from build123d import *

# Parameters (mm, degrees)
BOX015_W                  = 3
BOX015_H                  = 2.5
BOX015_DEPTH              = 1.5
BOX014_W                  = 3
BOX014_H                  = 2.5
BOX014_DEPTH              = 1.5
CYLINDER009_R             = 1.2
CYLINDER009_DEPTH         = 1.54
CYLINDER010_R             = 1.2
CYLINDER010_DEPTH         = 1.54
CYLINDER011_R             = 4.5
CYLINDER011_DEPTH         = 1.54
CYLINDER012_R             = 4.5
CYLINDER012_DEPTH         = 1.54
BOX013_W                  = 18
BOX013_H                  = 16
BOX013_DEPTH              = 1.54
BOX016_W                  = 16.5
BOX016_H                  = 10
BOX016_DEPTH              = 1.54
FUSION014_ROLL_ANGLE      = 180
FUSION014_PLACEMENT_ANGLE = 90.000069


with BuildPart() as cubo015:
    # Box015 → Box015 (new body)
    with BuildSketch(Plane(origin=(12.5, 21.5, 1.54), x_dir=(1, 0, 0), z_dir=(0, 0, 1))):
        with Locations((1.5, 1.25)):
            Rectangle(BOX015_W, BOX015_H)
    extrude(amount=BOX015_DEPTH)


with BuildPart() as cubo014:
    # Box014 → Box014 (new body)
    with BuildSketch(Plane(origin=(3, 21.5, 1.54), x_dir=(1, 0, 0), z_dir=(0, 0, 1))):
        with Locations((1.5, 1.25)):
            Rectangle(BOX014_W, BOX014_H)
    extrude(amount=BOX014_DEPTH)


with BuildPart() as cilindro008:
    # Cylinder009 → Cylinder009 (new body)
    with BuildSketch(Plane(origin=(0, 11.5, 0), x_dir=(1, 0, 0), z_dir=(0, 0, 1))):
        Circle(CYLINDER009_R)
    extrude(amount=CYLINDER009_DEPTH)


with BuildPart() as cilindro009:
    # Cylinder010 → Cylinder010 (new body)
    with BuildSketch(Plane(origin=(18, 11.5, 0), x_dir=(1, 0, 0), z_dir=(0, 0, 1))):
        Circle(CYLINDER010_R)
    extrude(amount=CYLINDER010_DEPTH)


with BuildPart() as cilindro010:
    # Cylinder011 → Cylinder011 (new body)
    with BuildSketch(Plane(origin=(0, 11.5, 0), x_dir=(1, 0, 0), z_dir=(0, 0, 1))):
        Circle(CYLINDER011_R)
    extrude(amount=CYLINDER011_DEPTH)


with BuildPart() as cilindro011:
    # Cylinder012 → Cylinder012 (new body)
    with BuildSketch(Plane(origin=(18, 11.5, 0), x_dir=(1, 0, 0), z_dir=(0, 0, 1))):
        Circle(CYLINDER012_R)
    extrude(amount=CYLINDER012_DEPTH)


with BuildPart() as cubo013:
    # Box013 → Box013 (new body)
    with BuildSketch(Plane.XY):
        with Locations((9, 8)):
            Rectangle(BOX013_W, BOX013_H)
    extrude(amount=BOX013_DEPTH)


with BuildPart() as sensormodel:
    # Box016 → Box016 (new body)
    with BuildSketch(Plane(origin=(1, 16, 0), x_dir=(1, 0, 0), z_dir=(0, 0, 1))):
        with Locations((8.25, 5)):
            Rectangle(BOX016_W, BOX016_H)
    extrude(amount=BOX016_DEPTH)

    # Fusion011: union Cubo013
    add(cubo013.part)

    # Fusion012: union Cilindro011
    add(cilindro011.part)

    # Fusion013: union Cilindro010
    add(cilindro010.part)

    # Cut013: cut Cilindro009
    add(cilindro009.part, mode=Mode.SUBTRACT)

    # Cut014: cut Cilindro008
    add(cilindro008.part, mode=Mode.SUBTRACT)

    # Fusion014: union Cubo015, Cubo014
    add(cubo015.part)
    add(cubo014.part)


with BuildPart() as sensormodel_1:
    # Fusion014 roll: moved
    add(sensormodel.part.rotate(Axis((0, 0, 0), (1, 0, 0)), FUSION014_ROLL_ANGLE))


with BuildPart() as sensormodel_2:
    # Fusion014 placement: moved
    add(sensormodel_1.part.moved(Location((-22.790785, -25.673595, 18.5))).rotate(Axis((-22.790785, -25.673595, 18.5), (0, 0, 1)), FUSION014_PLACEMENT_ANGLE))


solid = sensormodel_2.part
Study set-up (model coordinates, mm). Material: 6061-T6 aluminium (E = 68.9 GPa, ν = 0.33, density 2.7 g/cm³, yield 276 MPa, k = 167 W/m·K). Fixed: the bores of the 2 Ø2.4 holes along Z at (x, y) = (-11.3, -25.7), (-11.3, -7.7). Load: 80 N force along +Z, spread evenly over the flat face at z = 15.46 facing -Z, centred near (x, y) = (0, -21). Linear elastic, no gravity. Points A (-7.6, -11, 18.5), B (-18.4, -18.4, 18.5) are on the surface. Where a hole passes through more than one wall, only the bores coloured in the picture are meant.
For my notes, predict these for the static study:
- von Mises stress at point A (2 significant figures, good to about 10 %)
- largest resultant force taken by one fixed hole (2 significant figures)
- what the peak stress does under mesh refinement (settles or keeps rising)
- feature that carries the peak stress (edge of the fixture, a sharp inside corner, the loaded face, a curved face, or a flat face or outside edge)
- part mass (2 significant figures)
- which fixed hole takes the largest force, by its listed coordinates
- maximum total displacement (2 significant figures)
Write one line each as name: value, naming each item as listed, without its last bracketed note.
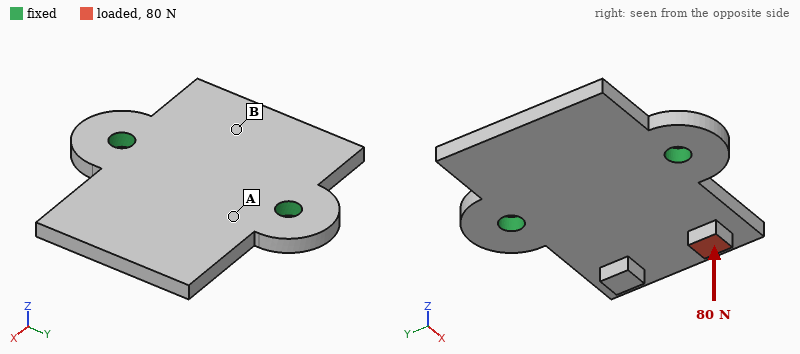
von Mises stress at point A: 73 MPa
largest resultant force taken by one fixed hole: 64 N
what the peak stress does under mesh refinement: keeps rising
feature that carries the peak stress: edge of the fixture
part mass: 2.2 g
which fixed hole takes the largest force, by its listed coordinates: (-11.3, -25.7)
maximum total displacement: 0.19 mm
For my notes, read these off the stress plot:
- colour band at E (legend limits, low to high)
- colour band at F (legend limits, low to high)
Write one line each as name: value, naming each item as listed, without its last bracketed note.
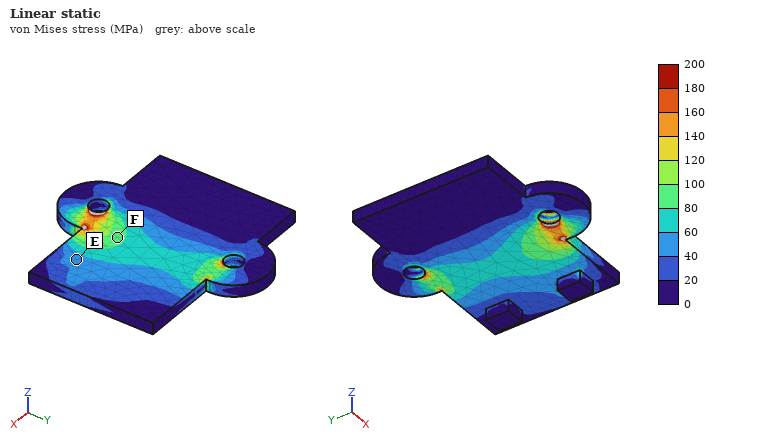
colour band at E: 40 to 60 MPa
colour band at F: 80 to 100 MPa
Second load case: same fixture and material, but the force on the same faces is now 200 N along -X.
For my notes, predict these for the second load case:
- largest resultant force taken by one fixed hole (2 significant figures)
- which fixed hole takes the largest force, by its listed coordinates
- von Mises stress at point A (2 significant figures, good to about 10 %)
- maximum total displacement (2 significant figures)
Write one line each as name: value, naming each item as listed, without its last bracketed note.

largest resultant force taken by one fixed hole: 150 N
which fixed hole takes the largest force, by its listed coordinates: (-11.3, -25.7)
von Mises stress at point A: 55 MPa
maximum total displacement: 0.15 mm
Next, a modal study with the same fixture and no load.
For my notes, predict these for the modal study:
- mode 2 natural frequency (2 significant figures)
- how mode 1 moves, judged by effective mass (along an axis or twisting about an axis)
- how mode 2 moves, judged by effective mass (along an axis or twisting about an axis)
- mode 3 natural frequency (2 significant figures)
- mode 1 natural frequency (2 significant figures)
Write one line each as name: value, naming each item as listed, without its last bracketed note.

mode 2 natural frequency: 9300 Hz
how mode 1 moves, judged by effective mass: along Z
how mode 2 moves, judged by effective mass: along Z
mode 3 natural frequency: 14 kHz
mode 1 natural frequency: 5400 Hz
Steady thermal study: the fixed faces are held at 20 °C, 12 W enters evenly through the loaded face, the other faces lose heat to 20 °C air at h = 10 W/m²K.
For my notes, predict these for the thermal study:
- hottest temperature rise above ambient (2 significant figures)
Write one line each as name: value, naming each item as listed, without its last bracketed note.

hottest temperature rise above ambient: 64 K
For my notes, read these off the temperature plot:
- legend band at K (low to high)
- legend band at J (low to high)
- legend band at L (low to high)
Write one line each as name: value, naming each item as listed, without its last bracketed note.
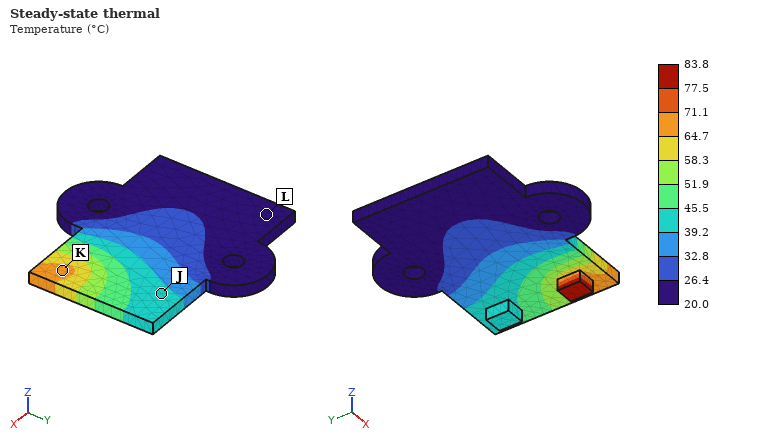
legend band at K: 64.7 to 71.1 °C
legend band at J: 39.2 to 45.5 °C
legend band at L: 20.0 to 26.4 °C
